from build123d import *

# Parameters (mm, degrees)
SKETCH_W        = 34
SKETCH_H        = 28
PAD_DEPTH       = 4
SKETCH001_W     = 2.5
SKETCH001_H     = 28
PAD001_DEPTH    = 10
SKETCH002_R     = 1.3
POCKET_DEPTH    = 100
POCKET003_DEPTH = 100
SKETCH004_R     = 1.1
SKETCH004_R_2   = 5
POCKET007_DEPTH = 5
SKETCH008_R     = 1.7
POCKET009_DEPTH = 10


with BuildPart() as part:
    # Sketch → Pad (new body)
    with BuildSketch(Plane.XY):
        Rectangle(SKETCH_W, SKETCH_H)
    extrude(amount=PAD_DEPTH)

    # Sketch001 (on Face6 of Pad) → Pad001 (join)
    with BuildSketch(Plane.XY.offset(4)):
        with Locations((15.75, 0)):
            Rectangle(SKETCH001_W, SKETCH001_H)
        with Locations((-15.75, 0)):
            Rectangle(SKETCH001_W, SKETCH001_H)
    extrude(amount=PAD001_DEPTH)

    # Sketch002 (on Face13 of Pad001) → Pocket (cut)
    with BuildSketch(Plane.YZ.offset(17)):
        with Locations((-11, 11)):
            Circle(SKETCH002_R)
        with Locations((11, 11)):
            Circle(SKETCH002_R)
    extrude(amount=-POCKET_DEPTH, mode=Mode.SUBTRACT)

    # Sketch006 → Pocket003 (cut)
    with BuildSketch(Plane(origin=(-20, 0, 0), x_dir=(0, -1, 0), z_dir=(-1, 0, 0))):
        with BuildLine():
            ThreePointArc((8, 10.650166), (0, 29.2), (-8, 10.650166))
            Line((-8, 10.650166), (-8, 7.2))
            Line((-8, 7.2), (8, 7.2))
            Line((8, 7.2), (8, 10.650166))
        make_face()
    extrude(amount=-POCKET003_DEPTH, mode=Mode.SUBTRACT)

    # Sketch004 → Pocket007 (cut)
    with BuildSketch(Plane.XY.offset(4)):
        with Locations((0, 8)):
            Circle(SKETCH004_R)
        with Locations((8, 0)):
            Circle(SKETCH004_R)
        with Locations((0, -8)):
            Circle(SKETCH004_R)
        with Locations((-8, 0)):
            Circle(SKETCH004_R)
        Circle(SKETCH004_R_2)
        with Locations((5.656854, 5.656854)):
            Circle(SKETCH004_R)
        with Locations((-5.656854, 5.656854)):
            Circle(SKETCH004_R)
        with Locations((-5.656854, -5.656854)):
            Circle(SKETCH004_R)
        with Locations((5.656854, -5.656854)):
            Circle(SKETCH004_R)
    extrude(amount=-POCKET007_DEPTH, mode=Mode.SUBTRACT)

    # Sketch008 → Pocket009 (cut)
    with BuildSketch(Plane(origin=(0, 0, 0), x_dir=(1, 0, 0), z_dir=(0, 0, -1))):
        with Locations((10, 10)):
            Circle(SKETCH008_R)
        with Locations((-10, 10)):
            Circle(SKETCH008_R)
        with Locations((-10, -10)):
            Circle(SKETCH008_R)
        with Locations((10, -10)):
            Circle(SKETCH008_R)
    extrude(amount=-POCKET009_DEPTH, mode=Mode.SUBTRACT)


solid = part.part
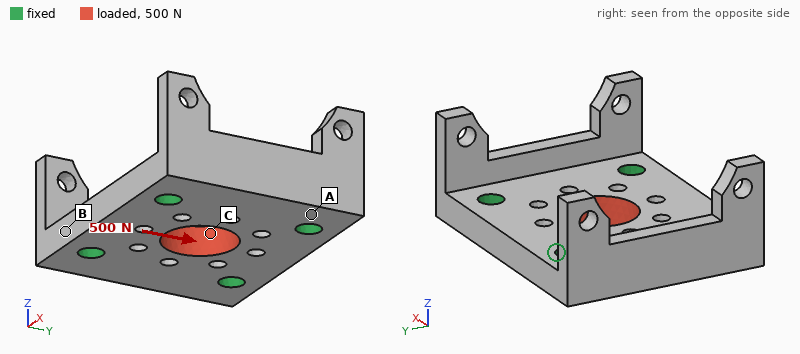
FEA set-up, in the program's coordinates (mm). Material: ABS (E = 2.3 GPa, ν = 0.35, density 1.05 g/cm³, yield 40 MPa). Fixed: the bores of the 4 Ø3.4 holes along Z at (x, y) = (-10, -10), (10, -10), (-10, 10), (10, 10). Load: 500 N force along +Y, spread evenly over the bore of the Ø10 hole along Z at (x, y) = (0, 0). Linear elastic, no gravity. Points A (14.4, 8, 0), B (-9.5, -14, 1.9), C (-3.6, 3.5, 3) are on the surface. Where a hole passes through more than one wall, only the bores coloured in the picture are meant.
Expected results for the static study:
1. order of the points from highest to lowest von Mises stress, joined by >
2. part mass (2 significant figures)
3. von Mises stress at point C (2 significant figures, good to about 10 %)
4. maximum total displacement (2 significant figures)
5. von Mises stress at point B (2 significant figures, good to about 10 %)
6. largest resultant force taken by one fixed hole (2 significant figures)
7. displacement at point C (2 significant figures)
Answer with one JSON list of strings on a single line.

["C > B > A", "4.2 g", "5.5 MPa", "32 µm", "3.2 MPa", "130 N", "28 µm"]
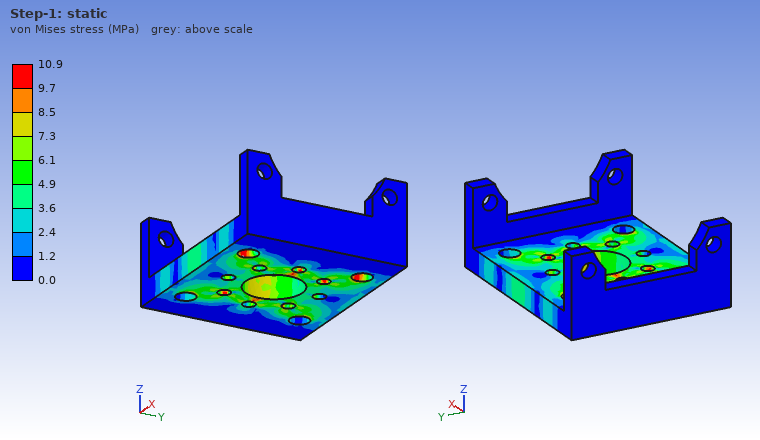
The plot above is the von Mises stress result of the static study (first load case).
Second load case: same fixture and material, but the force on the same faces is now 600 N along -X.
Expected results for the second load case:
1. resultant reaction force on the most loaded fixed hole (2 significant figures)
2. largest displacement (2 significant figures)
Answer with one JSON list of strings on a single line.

["150 N", "34 µm"]
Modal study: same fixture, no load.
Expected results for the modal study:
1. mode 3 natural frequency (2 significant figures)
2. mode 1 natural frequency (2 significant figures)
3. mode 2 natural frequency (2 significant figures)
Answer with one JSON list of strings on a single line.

["5500 Hz", "5300 Hz", "5300 Hz"]
